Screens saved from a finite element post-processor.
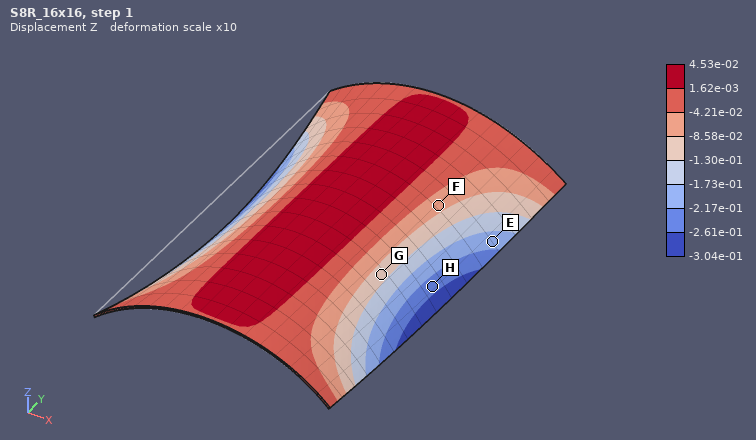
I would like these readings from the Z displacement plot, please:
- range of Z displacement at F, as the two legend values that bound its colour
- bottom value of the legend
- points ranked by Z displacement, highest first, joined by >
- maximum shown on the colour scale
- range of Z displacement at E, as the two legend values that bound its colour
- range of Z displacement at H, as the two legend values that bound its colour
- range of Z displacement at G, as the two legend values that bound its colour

-8.58e-02 to -4.21e-02
-3.04e-01
F > G > E > H
4.53e-02
-2.17e-01 to -1.73e-01
-2.61e-01 to -2.17e-01
-1.30e-01 to -8.58e-02
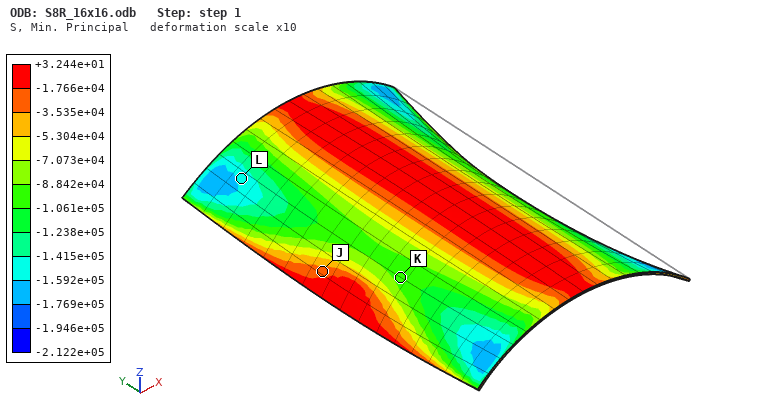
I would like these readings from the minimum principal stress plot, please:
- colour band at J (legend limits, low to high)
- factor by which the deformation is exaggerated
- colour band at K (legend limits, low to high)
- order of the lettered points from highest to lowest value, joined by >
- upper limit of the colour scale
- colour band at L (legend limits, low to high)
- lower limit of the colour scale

-3.535e+04 to -1.766e+04
10
-1.061e+05 to -8.842e+04
J > K > L
+3.244e+01
-1.592e+05 to -1.415e+05
-2.122e+05
